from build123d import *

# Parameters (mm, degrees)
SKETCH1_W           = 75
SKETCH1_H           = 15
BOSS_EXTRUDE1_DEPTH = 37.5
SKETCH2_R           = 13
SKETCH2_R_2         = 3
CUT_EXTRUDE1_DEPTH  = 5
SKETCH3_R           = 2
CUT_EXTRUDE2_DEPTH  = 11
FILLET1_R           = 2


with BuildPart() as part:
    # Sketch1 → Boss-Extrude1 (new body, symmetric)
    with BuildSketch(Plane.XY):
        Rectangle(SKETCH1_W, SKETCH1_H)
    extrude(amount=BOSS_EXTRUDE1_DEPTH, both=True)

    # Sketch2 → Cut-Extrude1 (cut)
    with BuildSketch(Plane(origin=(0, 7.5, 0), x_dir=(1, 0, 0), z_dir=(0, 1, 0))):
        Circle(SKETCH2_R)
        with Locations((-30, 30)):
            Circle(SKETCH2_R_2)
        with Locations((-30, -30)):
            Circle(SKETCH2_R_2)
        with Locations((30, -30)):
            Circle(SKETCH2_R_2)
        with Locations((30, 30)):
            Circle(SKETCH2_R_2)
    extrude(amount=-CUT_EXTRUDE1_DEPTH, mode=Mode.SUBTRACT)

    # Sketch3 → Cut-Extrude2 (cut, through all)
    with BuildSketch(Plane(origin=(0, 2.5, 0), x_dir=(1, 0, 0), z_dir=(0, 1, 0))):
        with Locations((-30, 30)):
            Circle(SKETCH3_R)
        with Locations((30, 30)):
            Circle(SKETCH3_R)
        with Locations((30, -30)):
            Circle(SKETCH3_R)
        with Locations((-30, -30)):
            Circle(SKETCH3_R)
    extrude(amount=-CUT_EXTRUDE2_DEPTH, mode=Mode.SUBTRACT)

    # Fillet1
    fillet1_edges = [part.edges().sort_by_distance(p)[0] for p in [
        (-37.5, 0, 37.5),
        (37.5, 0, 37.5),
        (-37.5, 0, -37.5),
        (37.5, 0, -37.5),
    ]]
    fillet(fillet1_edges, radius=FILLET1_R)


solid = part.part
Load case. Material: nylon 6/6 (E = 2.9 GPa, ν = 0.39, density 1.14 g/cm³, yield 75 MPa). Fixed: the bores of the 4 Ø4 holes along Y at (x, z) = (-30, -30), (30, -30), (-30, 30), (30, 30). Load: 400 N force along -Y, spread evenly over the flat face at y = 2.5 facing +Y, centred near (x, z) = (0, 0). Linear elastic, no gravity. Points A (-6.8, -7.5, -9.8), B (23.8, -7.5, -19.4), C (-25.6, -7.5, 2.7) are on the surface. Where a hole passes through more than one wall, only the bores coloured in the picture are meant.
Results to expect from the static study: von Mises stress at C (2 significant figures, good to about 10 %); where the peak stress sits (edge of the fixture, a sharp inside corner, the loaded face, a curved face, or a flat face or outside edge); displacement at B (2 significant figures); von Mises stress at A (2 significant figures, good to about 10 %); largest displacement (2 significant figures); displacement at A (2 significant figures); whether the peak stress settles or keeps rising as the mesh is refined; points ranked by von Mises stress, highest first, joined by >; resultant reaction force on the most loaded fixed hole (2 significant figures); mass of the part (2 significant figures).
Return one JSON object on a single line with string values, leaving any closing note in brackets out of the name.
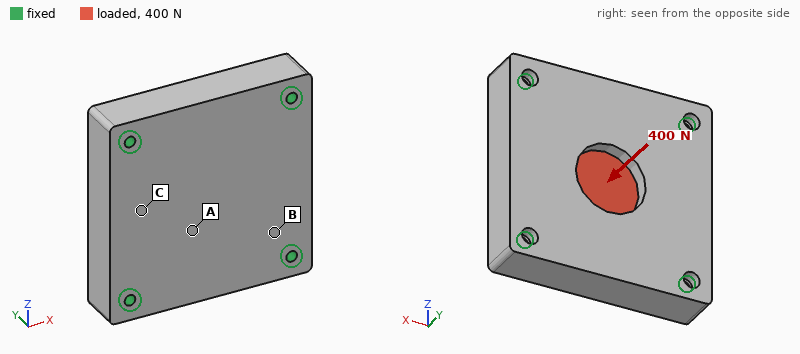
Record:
{"von Mises stress at C": "0.92 MPa", "where the peak stress sits": "edge of the fixture", "displacement at B": "16 µm", "von Mises stress at A": "1.9 MPa", "largest displacement": "50 µm", "displacement at A": "39 µm", "whether the peak stress settles or keeps rising as the mesh is refined": "keeps rising", "points ranked by von Mises stress, highest first, joined by >": "A > C > B", "resultant reaction force on the most loaded fixed hole": "110 N", "mass of the part": "92 g"}
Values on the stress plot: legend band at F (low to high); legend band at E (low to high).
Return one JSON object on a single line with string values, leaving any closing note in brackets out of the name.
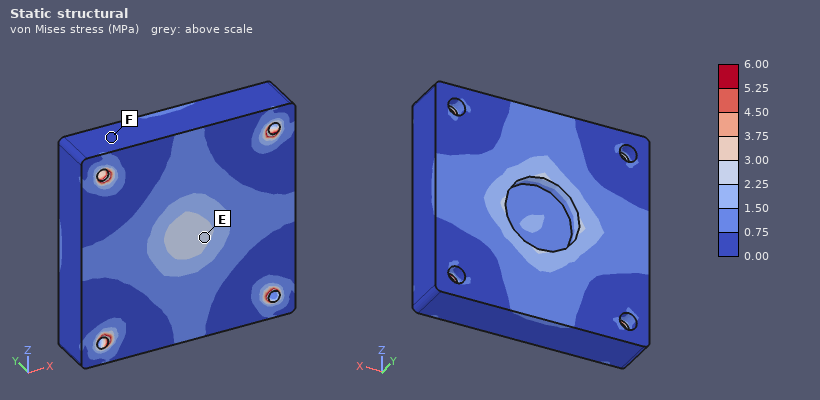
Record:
{"legend band at F": "0.00 to 0.75 MPa", "legend band at E": "2.25 to 3.00 MPa"}
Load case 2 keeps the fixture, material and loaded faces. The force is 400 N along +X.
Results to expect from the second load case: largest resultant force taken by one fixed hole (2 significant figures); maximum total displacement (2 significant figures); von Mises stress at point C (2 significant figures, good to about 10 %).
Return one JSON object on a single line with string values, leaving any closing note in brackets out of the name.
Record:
{"largest resultant force taken by one fixed hole": "110 N", "maximum total displacement": "12 µm", "von Mises stress at point C": "0.23 MPa"}
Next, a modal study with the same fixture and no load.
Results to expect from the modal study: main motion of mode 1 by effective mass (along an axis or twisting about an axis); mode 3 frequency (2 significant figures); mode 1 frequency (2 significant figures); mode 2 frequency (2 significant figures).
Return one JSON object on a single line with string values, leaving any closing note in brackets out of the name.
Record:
{"main motion of mode 1 by effective mass": "along Y", "mode 3 frequency": "4500 Hz", "mode 1 frequency": "2900 Hz", "mode 2 frequency": "4500 Hz"}
